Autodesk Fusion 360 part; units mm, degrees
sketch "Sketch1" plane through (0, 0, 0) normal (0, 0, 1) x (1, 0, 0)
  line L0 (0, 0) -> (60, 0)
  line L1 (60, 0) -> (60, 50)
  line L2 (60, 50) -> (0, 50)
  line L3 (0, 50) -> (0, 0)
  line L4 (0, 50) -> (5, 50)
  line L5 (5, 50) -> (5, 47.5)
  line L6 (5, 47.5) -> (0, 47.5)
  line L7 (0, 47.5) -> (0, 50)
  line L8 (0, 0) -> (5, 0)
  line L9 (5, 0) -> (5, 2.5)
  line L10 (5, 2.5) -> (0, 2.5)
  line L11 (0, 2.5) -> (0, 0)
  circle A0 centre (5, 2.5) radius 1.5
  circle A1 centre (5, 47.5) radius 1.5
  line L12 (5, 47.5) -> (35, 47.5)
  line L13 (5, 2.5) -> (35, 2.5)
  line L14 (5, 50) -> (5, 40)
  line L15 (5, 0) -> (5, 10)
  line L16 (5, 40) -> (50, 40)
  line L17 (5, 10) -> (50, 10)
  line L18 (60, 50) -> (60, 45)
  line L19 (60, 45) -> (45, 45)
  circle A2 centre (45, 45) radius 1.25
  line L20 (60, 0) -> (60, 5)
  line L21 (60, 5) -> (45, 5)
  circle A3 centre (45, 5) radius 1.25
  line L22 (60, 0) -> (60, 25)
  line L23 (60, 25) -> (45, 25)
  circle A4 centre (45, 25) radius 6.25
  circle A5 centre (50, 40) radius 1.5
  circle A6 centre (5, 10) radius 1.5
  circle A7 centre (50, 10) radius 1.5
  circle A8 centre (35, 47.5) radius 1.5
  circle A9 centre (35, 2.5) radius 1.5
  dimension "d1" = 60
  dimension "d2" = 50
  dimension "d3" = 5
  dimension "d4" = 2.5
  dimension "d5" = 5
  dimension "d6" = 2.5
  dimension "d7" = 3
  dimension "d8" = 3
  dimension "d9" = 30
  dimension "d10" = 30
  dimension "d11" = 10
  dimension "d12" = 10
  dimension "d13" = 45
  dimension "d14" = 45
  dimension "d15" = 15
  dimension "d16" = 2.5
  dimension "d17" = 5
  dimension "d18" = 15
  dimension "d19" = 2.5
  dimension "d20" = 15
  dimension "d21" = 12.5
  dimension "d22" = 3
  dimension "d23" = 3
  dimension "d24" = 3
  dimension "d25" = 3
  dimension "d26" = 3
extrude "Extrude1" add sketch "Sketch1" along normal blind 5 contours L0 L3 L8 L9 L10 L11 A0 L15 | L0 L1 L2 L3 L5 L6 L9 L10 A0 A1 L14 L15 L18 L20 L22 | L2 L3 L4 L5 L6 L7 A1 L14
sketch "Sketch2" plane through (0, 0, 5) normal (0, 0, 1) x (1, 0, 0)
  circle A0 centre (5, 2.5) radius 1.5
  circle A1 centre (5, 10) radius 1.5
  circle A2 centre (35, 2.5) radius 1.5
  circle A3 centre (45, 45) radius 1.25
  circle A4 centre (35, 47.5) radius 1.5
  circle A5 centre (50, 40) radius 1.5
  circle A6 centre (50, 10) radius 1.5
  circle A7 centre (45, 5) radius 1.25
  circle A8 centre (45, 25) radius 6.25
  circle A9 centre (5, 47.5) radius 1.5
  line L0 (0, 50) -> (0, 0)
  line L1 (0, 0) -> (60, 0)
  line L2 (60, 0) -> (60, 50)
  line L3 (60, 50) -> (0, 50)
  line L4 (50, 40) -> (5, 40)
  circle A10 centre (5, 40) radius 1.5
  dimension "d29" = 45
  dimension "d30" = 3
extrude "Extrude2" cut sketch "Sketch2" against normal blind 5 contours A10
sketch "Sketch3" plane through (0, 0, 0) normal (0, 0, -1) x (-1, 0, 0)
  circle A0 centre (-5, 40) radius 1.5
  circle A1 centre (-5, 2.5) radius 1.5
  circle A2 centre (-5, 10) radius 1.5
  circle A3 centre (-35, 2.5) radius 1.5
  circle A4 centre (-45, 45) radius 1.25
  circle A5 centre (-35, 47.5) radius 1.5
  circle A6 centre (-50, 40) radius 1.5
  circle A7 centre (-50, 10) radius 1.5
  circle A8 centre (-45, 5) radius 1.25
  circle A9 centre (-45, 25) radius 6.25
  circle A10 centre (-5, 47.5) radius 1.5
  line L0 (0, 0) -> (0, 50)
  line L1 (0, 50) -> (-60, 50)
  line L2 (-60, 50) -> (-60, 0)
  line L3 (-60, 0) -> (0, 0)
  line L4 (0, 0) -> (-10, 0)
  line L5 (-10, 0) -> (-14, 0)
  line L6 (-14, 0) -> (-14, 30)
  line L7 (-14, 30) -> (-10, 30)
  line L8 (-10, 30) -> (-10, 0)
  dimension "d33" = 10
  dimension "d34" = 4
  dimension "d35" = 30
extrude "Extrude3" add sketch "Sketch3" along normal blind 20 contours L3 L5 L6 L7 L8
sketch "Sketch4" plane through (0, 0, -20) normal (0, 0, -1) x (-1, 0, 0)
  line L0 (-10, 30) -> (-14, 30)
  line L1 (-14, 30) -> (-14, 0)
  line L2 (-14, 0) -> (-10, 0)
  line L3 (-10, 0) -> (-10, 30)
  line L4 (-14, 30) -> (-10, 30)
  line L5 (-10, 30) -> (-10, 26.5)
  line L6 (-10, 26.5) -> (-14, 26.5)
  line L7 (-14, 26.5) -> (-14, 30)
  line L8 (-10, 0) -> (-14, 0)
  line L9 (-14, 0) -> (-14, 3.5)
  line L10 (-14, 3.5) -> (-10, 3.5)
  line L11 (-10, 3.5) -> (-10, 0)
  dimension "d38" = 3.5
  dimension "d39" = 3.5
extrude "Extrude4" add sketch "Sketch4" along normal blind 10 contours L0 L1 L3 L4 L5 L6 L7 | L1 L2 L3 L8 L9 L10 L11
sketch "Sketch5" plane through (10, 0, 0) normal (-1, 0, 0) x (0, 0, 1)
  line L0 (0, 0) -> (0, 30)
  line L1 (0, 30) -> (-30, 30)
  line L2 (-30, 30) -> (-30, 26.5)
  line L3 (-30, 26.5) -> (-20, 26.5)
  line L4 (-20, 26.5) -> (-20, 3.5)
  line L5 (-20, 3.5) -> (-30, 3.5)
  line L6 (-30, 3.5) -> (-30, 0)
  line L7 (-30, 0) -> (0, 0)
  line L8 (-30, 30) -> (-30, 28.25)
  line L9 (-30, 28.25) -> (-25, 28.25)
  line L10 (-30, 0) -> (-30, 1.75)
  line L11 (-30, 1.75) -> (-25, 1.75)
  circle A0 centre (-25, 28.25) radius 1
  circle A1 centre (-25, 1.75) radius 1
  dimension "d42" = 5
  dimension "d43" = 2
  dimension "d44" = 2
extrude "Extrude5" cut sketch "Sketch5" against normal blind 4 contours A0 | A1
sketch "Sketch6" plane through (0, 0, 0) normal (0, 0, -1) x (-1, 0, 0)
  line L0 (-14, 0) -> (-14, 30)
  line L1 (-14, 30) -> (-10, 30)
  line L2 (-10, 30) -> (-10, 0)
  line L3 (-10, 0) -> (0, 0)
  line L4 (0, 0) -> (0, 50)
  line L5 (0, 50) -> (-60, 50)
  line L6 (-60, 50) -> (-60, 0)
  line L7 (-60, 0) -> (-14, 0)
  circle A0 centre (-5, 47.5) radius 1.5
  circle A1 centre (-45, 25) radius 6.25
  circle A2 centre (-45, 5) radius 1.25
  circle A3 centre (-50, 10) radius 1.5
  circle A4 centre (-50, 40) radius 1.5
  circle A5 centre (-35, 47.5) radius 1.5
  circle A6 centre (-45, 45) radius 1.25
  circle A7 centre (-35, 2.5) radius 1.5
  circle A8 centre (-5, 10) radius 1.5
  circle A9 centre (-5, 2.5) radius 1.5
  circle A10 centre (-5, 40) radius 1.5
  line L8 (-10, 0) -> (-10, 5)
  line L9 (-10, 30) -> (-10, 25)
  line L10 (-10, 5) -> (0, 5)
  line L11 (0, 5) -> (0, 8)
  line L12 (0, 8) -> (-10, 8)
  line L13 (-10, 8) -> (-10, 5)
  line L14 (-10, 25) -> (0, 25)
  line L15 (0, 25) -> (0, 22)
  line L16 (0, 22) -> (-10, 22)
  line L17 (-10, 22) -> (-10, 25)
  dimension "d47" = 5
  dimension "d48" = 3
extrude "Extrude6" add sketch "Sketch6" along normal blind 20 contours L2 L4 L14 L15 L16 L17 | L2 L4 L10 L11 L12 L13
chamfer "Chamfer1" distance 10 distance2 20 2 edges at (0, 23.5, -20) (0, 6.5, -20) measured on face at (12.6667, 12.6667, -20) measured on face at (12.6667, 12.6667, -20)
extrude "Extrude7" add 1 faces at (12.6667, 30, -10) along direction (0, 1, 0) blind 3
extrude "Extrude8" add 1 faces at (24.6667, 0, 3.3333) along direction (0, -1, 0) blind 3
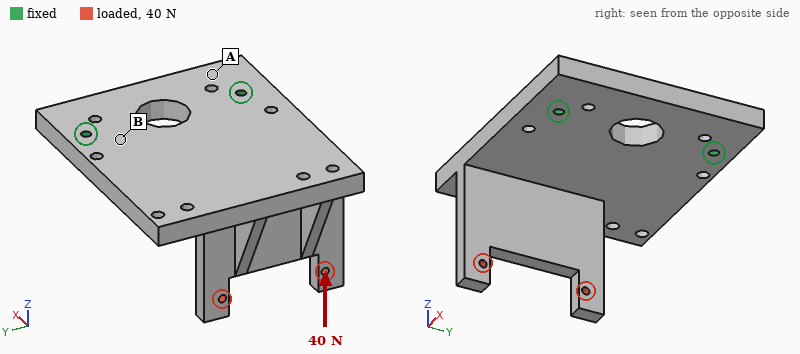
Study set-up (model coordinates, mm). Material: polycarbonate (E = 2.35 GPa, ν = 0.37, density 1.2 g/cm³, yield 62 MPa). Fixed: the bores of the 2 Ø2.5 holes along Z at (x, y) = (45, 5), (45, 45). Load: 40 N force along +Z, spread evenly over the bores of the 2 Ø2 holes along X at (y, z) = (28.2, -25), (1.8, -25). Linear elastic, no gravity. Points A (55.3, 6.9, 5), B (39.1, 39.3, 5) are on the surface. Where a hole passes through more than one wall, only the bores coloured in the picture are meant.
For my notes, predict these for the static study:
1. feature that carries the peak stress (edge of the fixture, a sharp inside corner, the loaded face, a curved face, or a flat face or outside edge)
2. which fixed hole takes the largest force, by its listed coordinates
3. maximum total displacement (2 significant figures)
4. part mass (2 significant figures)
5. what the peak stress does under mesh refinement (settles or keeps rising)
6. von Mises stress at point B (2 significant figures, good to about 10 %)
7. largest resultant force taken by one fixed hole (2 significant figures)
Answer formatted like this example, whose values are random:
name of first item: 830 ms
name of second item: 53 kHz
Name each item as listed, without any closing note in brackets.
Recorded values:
feature that carries the peak stress: edge of the fixture
which fixed hole takes the largest force, by its listed coordinates: (45, 5)
maximum total displacement: 1.0 mm
part mass: 23 g
what the peak stress does under mesh refinement: keeps rising
von Mises stress at point B: 5.1 MPa
largest resultant force taken by one fixed hole: 30 N
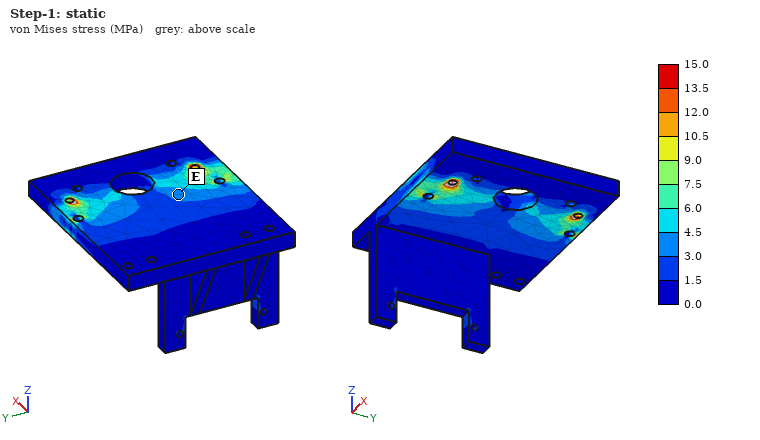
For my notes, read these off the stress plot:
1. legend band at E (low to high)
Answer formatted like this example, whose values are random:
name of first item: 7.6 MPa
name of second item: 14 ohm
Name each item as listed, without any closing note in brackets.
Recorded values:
legend band at E: 3.0 to 4.5 MPa
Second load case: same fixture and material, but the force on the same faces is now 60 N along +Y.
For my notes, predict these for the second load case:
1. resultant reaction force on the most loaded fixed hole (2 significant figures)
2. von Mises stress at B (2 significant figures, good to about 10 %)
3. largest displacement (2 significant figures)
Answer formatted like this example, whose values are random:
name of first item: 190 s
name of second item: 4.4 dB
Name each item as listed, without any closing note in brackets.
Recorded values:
resultant reaction force on the most loaded fixed hole: 70 N
von Mises stress at B: 3.4 MPa
largest displacement: 0.82 mm
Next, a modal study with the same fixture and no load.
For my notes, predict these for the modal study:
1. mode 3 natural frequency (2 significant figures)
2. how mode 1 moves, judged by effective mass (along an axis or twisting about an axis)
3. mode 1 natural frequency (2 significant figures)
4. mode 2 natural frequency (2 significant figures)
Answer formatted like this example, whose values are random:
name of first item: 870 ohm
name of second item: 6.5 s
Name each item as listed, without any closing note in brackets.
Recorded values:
mode 3 natural frequency: 1400 Hz
how mode 1 moves, judged by effective mass: along Z
mode 1 natural frequency: 330 Hz
mode 2 natural frequency: 820 Hz
